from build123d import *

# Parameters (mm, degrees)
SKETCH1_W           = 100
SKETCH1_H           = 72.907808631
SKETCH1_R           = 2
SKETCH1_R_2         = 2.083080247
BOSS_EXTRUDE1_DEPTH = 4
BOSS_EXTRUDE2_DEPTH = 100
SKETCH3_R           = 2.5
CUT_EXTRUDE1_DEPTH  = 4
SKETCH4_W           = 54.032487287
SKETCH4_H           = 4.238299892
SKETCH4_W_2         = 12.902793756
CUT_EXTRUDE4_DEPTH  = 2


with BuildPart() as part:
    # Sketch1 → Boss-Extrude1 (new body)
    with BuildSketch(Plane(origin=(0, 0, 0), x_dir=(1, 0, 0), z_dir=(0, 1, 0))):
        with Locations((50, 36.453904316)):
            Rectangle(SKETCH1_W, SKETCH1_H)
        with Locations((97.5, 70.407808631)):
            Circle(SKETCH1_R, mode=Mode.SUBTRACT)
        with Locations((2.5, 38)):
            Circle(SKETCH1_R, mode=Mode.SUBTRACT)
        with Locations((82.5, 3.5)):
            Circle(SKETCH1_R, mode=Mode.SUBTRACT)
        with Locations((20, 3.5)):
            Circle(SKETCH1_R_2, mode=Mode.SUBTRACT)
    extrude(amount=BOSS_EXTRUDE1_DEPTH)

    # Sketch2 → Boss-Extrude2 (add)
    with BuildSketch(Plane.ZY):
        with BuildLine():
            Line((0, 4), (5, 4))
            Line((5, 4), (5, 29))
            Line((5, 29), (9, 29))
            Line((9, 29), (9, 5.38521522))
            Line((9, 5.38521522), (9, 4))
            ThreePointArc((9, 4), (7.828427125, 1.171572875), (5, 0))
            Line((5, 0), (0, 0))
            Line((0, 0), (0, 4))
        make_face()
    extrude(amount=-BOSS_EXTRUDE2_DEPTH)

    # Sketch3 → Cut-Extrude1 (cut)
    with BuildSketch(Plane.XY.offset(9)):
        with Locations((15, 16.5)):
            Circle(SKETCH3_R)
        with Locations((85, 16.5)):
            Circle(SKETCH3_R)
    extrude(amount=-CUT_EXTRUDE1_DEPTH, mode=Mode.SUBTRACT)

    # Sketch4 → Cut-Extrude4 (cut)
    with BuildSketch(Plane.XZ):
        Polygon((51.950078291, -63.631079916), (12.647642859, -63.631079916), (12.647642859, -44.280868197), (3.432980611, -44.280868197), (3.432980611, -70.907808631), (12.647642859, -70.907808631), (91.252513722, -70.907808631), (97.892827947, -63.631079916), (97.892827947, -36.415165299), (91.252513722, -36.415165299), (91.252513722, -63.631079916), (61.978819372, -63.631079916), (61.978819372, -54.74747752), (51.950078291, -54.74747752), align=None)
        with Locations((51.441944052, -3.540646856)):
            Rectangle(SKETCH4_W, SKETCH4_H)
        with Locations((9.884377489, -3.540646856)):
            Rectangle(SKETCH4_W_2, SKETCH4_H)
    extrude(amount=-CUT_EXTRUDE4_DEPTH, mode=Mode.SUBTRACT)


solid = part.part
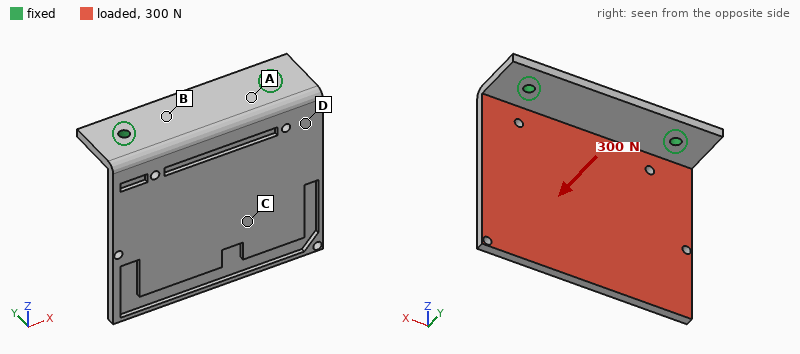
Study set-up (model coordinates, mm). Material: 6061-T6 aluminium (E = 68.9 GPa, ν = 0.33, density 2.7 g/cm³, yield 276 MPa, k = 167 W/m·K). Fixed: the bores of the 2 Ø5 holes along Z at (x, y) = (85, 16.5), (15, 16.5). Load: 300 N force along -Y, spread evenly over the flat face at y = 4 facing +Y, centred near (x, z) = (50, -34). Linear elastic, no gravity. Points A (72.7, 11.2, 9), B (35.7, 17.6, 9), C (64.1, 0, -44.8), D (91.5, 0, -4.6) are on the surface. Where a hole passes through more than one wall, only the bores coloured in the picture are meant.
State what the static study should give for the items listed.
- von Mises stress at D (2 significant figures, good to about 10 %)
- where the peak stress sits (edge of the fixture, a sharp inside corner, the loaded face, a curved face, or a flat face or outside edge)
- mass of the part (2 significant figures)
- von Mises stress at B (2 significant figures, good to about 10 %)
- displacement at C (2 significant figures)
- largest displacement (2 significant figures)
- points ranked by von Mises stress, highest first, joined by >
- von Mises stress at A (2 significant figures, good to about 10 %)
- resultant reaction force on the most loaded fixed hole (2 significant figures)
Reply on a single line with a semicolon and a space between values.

49 MPa; a curved face; 110 g; 19 MPa; 0.72 mm; 1.2 mm; D > A > B > C; 35 MPa; 170 N
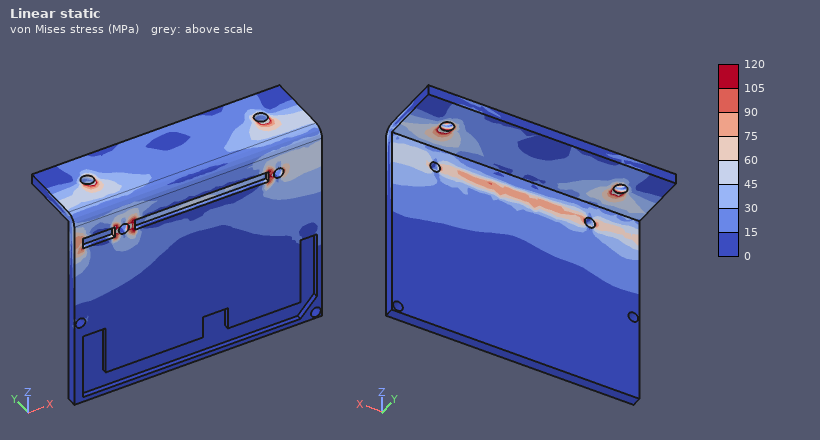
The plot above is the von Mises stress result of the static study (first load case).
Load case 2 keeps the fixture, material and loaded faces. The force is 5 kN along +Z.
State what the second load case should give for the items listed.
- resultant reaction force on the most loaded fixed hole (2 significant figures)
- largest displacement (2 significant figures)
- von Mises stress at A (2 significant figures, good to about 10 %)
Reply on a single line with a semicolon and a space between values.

2.5 kN; 0.62 mm; 86 MPa
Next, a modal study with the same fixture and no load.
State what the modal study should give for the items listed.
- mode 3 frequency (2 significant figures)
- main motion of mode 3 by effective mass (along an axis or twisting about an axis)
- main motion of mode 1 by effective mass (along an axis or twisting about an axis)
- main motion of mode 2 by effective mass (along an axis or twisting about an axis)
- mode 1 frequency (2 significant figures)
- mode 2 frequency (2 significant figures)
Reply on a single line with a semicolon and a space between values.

2100 Hz; along X; along Y; twisting about Z; 370 Hz; 960 Hz
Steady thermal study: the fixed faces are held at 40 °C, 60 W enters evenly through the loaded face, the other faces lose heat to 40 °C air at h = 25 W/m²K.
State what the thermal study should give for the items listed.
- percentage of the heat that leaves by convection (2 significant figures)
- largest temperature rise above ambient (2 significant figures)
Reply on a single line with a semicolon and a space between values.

20 %; 51 K
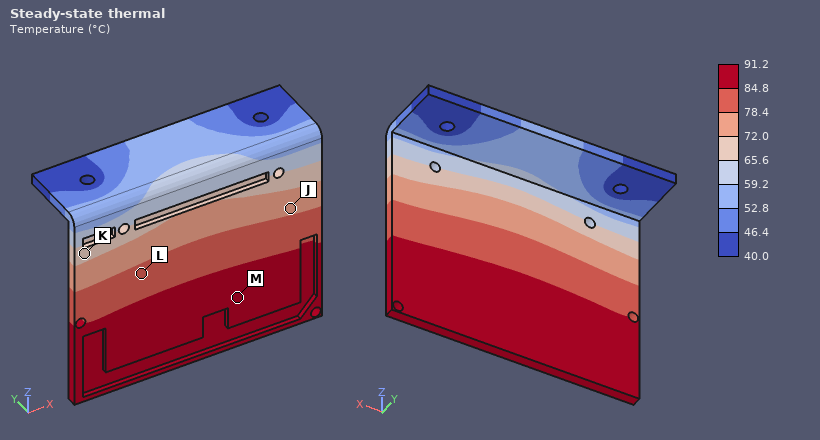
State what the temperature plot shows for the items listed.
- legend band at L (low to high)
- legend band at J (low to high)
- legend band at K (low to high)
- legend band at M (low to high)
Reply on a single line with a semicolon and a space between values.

78.4 to 84.8 °C; 72.0 to 78.4 °C; 65.6 to 72.0 °C; 84.8 to 91.2 °C
